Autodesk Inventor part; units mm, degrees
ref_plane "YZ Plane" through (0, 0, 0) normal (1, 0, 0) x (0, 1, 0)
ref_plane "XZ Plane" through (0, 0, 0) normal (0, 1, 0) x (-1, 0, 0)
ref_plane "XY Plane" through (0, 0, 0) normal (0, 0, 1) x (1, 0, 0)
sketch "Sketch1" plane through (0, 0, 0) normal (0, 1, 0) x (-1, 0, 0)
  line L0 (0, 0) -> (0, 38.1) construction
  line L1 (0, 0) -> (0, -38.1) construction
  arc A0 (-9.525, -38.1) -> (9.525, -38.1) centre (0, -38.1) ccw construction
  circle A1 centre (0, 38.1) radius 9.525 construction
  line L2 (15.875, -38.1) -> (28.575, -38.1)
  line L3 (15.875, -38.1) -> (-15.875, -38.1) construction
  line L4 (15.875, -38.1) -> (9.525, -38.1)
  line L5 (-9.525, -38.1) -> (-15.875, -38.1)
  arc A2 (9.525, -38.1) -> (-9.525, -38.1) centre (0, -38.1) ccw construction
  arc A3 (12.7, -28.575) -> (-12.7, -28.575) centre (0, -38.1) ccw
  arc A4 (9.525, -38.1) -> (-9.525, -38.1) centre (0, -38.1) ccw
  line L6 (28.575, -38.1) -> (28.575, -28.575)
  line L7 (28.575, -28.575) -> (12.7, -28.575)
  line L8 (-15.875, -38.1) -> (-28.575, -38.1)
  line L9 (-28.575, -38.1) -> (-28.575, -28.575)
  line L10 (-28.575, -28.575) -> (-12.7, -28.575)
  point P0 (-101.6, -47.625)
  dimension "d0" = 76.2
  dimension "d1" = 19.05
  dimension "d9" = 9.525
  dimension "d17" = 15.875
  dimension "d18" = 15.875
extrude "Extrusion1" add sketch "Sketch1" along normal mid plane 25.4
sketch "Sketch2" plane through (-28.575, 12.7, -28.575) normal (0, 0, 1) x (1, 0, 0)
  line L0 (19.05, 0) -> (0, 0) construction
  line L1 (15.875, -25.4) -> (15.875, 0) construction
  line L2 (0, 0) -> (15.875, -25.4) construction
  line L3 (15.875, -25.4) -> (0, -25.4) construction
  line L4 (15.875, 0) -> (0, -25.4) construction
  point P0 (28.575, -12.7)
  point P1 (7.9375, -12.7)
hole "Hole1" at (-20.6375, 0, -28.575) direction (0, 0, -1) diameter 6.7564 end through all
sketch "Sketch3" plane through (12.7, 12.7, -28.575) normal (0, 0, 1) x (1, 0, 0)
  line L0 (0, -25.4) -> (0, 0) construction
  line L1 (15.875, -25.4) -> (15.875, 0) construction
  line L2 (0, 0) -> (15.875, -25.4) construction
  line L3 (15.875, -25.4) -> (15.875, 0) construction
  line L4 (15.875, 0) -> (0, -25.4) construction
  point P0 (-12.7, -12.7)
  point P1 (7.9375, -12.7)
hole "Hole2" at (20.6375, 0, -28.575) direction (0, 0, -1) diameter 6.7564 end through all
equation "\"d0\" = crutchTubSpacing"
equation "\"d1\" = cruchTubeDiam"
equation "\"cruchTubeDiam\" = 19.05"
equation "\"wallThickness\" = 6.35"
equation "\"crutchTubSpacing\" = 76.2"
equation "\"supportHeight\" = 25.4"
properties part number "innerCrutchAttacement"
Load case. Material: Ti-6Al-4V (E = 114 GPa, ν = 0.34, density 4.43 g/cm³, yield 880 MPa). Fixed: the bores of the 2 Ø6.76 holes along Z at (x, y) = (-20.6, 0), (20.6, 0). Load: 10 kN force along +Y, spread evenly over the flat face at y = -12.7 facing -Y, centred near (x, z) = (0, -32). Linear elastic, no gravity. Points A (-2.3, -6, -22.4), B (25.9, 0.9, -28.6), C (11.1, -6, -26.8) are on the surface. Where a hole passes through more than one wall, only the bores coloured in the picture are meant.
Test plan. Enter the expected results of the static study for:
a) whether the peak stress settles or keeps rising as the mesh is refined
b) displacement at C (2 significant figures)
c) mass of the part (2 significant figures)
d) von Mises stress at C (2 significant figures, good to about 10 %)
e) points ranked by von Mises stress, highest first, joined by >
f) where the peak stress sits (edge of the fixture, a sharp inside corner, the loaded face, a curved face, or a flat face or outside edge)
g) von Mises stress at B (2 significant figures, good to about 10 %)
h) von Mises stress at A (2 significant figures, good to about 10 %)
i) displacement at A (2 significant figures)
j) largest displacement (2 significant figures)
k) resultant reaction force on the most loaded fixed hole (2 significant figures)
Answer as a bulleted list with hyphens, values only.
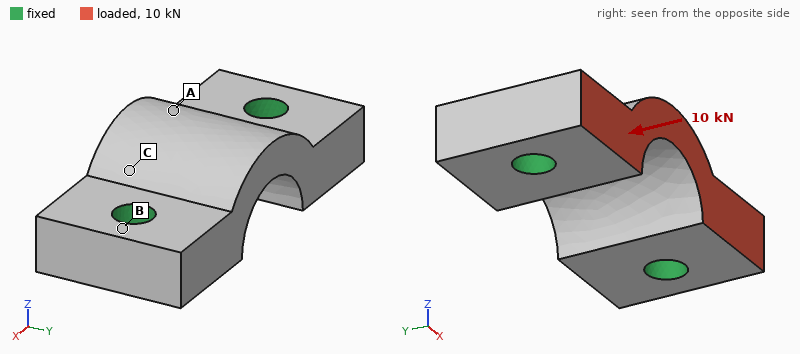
- keeps rising
- 8.8 µm
- 55 g
- 36 MPa
- C > A > B
- edge of the fixture
- 9.4 MPa
- 20 MPa
- 14 µm
- 18 µm
- 5.0 kN
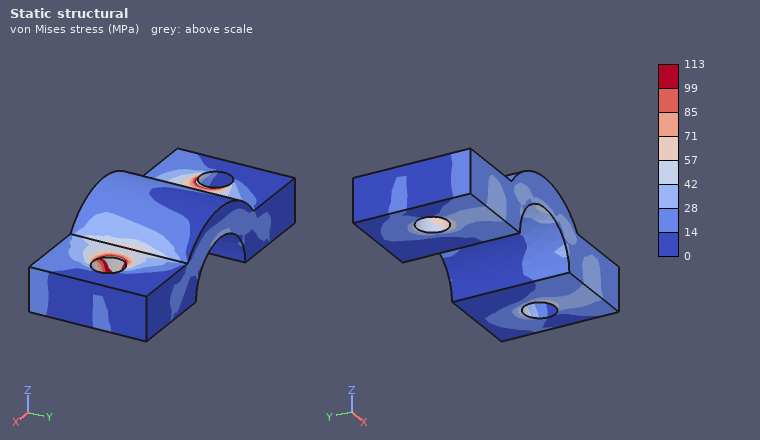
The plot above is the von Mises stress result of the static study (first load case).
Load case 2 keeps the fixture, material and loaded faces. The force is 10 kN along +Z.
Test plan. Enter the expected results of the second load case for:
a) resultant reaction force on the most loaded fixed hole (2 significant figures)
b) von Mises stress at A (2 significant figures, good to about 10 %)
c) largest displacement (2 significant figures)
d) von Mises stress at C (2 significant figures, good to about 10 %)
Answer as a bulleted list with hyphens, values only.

- 5.2 kN
- 55 MPa
- 46 µm
- 53 MPa
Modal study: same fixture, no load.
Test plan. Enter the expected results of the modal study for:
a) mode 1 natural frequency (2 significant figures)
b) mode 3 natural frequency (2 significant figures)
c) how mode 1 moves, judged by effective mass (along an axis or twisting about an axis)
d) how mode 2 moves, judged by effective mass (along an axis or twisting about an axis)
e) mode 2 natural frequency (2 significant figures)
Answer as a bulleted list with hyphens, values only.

- 19 kHz
- 33 kHz
- along Y
- along Z
- 27 kHz
